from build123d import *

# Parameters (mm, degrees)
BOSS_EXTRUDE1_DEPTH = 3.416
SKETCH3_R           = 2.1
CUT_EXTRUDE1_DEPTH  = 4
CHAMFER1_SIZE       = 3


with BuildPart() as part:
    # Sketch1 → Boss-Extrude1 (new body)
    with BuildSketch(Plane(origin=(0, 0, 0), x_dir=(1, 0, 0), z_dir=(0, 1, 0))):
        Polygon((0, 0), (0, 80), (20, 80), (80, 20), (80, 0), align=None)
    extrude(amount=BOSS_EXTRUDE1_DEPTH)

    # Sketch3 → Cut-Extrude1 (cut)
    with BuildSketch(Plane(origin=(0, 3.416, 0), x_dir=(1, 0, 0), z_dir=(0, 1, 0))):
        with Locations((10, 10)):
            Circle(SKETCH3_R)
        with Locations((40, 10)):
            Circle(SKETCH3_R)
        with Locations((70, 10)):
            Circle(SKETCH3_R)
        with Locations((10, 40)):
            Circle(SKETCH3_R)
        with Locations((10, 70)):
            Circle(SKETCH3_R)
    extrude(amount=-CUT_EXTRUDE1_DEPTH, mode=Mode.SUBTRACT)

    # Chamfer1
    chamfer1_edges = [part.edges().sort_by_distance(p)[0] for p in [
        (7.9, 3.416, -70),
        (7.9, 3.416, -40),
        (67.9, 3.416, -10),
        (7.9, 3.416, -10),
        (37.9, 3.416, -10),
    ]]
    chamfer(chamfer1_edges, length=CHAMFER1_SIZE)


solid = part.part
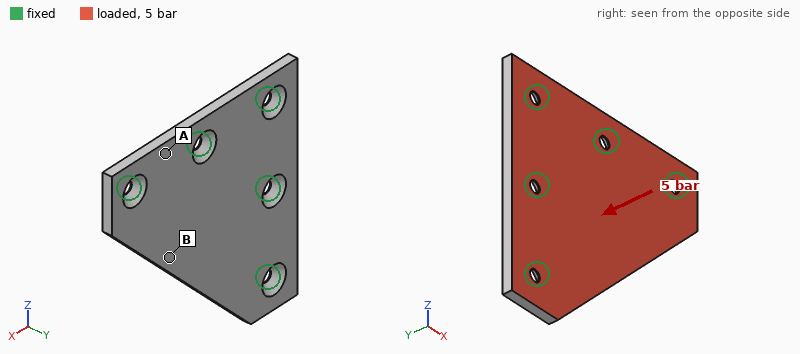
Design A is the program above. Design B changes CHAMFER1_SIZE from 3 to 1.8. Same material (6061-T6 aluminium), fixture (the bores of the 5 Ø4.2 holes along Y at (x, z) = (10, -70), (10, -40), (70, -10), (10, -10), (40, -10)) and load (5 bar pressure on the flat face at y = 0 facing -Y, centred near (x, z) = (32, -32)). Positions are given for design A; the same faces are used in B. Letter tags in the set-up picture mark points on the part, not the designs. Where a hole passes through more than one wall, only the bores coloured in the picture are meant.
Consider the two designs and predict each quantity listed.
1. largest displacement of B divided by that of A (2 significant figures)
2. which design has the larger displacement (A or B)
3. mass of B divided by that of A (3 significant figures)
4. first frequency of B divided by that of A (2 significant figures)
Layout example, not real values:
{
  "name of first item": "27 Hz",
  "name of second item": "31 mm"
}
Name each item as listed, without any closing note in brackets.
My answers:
{
  "largest displacement of B divided by that of A": "0.69",
  "which design has the larger displacement": "A",
  "mass of B divided by that of A": "1.02",
  "first frequency of B divided by that of A": "1.2"
}
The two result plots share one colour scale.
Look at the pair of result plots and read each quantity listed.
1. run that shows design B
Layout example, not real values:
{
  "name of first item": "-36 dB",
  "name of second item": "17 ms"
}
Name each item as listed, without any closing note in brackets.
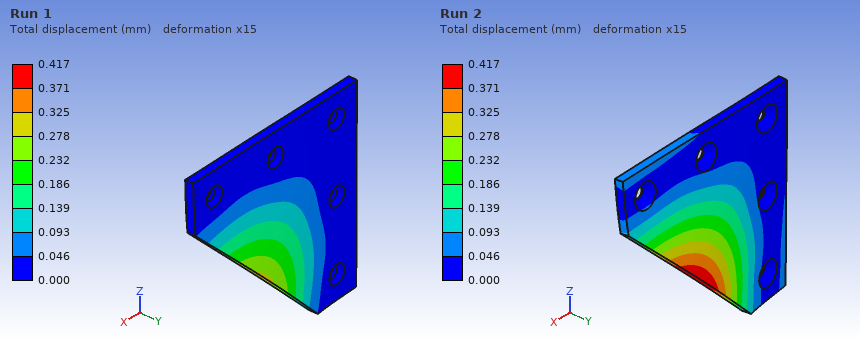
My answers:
{
  "run that shows design B": "Run 1"
}
